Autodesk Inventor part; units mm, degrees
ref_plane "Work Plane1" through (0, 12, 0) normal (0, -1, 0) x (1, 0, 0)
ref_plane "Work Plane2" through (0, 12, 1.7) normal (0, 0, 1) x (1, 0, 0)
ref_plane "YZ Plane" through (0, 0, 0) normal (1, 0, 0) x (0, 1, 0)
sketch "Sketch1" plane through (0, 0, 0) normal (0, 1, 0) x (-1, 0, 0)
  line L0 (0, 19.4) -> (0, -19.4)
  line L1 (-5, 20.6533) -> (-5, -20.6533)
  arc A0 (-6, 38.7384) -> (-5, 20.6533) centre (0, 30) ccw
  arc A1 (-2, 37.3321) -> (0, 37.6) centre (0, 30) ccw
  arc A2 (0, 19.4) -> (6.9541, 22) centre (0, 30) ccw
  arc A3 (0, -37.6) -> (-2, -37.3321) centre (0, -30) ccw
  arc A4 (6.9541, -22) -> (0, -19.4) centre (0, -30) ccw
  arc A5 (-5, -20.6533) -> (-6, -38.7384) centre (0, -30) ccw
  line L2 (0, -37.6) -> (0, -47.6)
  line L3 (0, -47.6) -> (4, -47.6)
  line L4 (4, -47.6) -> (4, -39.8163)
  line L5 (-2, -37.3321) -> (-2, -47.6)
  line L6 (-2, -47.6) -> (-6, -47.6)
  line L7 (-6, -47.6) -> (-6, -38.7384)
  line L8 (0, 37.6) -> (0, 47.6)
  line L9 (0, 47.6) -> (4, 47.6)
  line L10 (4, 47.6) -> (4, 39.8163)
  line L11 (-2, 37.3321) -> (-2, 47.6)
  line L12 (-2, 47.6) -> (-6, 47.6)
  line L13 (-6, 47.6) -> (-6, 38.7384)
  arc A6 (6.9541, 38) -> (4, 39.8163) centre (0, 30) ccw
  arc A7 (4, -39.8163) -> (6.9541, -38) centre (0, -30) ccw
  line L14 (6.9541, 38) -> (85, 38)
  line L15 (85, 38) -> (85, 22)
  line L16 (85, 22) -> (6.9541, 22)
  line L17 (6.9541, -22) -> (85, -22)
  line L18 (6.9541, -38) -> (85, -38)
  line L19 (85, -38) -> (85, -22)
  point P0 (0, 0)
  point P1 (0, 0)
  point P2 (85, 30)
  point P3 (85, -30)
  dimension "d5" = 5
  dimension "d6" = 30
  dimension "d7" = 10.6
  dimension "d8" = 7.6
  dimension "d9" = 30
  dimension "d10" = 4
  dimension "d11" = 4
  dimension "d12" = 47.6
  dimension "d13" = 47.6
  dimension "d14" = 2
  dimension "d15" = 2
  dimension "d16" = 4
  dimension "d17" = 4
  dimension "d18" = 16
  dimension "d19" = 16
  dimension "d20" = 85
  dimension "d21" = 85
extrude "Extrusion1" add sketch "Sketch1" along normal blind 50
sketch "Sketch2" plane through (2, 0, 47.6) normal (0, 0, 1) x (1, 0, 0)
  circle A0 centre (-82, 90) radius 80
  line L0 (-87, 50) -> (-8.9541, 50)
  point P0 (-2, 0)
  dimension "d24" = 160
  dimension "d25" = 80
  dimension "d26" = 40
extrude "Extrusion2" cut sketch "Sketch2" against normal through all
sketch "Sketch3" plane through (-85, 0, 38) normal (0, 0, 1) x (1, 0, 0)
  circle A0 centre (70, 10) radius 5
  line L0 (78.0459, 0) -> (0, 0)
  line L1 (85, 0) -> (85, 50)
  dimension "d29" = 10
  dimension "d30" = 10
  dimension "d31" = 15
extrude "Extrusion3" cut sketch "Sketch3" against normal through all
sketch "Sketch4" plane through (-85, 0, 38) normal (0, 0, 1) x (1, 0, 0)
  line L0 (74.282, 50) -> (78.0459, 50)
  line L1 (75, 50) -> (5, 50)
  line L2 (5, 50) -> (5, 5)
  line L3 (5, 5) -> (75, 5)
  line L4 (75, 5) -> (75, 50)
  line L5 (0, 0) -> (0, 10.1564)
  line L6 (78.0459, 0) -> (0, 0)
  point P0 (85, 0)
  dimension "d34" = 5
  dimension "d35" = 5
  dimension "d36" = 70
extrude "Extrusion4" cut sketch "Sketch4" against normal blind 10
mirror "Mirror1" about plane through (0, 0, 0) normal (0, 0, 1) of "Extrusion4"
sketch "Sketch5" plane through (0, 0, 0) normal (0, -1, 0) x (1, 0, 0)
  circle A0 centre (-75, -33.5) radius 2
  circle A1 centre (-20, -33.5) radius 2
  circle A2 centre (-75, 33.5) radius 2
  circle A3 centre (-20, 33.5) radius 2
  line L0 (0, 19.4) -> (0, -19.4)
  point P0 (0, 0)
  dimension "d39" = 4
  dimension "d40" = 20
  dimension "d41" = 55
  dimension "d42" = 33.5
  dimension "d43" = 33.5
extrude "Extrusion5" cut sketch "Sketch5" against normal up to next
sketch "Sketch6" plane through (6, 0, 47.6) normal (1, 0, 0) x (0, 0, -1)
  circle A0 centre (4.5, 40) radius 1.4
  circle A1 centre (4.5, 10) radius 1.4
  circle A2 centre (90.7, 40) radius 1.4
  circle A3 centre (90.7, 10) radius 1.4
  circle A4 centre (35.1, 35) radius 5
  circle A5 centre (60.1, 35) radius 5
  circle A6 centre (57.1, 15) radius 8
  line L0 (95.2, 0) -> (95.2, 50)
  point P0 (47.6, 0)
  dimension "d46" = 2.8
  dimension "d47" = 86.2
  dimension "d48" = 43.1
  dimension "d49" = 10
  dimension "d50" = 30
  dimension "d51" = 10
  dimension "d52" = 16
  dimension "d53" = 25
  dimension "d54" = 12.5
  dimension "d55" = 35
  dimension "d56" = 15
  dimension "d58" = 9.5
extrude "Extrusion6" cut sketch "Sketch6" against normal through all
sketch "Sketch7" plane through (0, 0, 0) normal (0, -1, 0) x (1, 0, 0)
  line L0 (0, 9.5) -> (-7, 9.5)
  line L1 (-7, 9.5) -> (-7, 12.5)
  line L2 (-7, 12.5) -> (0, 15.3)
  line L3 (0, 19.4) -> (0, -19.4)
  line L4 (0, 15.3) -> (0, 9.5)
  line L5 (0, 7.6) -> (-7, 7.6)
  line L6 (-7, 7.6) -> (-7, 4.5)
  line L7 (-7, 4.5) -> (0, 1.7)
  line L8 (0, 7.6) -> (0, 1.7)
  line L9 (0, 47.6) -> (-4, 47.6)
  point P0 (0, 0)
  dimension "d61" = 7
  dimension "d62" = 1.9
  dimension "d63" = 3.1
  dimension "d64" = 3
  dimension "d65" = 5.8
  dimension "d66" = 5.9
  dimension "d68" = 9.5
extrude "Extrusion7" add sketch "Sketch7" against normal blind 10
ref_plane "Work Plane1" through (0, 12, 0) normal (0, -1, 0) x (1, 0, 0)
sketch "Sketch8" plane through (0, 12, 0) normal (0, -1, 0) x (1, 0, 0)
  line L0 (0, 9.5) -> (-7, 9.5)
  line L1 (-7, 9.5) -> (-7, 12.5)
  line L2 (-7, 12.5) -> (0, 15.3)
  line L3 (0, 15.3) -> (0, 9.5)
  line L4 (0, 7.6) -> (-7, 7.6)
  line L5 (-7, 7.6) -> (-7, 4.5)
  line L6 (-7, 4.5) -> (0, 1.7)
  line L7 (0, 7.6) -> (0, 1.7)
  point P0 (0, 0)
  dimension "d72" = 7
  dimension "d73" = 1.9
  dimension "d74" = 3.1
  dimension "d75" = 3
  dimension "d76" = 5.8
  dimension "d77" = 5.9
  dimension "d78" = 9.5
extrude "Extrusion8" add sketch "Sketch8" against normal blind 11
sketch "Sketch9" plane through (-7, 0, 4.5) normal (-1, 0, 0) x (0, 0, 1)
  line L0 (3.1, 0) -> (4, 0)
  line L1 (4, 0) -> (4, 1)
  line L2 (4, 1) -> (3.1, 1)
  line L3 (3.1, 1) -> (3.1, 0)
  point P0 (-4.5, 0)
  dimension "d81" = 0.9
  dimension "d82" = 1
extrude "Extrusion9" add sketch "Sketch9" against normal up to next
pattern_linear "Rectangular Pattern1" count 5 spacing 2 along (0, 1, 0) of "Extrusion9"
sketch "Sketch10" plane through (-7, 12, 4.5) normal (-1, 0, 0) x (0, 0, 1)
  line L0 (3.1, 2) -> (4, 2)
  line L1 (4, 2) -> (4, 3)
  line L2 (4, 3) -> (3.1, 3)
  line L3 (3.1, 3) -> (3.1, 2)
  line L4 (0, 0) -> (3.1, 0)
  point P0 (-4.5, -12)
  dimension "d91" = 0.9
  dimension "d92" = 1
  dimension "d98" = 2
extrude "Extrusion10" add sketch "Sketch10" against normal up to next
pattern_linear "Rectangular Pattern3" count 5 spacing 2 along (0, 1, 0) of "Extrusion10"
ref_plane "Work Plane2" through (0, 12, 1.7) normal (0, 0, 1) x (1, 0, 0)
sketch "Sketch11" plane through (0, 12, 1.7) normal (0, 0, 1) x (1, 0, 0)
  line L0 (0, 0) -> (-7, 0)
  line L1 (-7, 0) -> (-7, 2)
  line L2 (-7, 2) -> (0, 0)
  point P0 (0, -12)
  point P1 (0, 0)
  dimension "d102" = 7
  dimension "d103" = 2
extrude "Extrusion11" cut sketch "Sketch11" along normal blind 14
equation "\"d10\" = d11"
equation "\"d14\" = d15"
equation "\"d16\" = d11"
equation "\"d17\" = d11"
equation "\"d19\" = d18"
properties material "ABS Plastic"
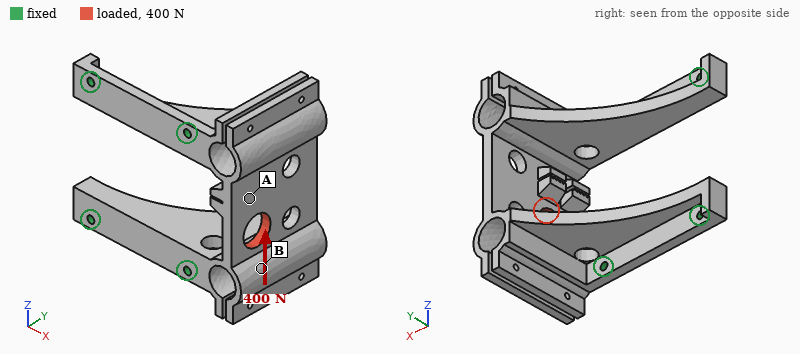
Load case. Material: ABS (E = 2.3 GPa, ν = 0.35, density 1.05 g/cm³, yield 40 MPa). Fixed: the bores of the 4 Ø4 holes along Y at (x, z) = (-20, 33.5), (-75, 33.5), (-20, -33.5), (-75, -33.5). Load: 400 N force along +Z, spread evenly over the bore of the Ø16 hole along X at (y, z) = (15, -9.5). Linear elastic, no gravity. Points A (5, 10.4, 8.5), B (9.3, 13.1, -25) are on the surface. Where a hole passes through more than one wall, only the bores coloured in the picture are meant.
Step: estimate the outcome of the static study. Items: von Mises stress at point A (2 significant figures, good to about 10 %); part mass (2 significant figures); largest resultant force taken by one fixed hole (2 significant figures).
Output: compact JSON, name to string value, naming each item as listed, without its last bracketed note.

{"von Mises stress at point A": "3.8 MPa", "part mass": "61 g", "largest resultant force taken by one fixed hole": "290 N"}
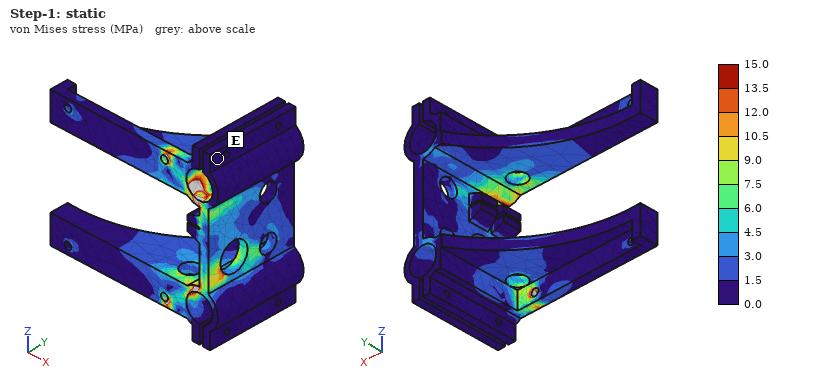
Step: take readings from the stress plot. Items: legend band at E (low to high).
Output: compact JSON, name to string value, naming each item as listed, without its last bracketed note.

{"legend band at E": "0.0 to 1.5 MPa"}
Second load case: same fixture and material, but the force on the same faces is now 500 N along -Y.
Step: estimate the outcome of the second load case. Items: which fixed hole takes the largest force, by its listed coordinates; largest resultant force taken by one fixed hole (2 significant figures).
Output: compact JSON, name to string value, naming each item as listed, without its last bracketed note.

{"which fixed hole takes the largest force, by its listed coordinates": "(-20, -33.5)", "largest resultant force taken by one fixed hole": "450 N"}
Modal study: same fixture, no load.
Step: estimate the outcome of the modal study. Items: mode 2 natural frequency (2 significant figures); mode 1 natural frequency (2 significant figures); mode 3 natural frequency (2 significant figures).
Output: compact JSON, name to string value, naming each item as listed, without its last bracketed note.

{"mode 2 natural frequency": "690 Hz", "mode 1 natural frequency": "670 Hz", "mode 3 natural frequency": "810 Hz"}
